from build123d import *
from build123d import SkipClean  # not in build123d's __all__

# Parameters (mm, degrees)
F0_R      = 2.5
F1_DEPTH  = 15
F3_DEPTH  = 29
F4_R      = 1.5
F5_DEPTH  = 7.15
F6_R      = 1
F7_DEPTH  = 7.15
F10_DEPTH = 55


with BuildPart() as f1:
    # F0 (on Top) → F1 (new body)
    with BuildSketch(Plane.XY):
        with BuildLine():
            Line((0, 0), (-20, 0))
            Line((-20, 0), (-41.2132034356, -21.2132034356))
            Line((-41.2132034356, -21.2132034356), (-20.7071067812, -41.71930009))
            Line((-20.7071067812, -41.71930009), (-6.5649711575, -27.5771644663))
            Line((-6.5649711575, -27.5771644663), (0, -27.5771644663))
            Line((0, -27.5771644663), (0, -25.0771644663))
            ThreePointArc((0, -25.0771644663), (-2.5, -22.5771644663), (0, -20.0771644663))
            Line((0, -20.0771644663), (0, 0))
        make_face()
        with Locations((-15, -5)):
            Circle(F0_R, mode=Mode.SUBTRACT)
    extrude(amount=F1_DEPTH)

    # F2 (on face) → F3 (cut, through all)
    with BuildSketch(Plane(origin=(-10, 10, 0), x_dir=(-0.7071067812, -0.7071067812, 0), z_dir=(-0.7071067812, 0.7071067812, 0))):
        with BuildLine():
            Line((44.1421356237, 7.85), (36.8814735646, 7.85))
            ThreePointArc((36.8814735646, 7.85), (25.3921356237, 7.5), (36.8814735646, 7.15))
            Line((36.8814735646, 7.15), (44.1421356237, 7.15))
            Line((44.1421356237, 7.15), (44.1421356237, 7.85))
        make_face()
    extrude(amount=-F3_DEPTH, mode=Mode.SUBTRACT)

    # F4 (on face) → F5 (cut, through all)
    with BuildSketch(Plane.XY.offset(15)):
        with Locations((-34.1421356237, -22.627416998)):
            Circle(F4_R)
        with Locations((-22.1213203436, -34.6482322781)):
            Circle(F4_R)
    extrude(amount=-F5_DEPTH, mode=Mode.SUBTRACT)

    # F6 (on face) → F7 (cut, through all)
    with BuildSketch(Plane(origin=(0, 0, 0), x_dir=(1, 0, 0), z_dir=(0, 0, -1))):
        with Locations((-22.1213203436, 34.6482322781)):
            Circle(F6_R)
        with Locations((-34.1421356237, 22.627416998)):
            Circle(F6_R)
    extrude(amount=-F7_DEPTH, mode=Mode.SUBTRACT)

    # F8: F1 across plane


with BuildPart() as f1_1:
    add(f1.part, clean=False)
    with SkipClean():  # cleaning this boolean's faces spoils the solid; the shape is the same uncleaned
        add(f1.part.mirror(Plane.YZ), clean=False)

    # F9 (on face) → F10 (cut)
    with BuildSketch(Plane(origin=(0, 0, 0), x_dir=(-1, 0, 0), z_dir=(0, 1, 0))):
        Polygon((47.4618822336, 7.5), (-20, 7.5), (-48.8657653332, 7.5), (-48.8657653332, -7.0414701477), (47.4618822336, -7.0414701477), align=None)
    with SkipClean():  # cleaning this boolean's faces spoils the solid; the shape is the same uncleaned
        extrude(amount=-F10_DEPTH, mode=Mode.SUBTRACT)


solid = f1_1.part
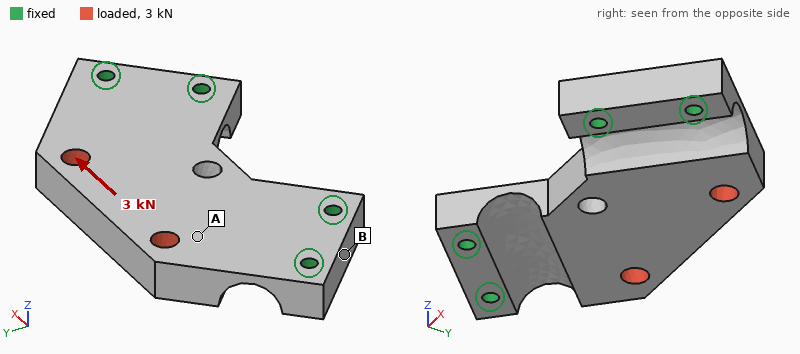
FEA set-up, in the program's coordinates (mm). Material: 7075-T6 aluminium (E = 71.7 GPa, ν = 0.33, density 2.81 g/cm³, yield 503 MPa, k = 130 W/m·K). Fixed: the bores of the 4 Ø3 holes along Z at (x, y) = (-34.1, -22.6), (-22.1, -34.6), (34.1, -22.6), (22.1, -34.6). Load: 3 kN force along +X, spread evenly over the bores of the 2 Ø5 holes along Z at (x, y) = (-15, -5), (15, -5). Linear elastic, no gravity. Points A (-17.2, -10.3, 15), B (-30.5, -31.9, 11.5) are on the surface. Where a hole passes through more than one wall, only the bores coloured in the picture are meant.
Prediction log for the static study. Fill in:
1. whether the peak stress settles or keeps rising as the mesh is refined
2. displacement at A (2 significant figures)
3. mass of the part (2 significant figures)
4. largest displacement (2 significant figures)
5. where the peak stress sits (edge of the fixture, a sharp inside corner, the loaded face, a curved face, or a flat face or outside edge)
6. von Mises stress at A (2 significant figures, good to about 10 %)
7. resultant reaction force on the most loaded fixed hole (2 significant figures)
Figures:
keeps rising
12 µm
35 g
18 µm
edge of the fixture
26 MPa
1.3 kN
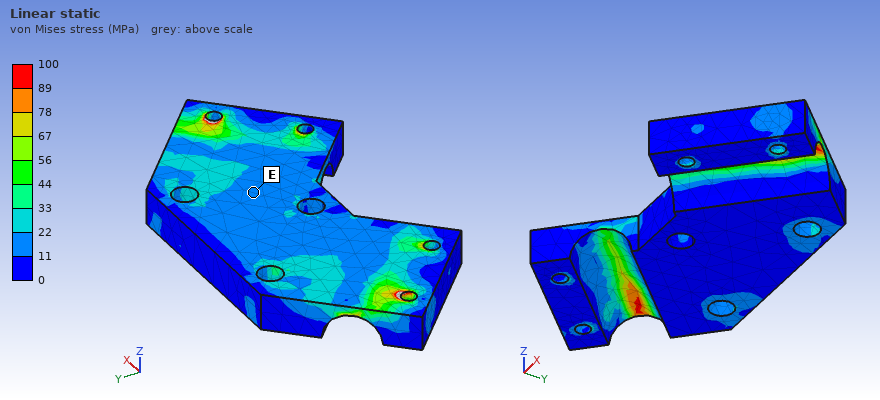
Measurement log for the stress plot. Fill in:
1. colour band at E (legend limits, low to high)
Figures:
11 to 22 MPa
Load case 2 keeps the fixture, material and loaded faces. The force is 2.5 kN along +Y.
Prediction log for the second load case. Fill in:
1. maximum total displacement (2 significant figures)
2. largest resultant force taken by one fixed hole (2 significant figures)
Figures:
0.13 mm
1.1 kN
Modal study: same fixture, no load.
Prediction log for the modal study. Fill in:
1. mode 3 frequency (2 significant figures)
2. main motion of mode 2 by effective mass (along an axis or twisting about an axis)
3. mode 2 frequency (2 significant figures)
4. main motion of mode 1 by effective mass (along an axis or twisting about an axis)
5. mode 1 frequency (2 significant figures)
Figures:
11 kHz
twisting about Y
9400 Hz
along Z
2700 Hz
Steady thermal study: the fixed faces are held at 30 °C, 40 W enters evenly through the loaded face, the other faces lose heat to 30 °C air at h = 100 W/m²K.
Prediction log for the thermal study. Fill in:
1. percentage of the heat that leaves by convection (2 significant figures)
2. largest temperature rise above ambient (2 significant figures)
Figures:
26 %
37 K
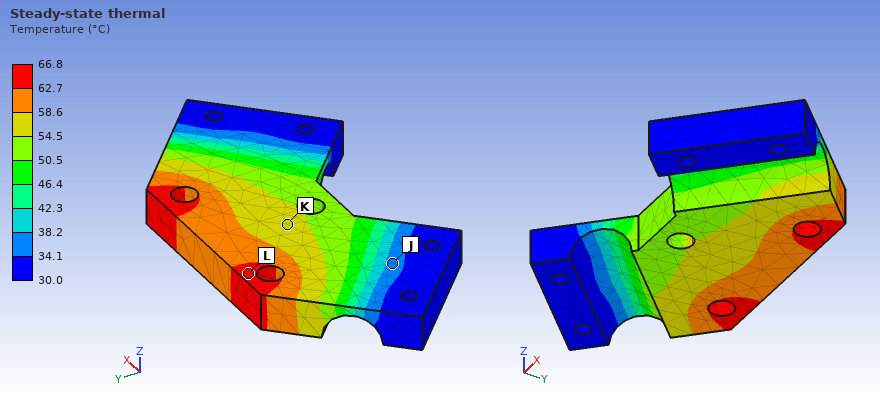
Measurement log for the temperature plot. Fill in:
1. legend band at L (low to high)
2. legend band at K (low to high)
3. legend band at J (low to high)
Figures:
62.7 to 66.8 °C
54.5 to 58.6 °C
34.1 to 38.2 °C
